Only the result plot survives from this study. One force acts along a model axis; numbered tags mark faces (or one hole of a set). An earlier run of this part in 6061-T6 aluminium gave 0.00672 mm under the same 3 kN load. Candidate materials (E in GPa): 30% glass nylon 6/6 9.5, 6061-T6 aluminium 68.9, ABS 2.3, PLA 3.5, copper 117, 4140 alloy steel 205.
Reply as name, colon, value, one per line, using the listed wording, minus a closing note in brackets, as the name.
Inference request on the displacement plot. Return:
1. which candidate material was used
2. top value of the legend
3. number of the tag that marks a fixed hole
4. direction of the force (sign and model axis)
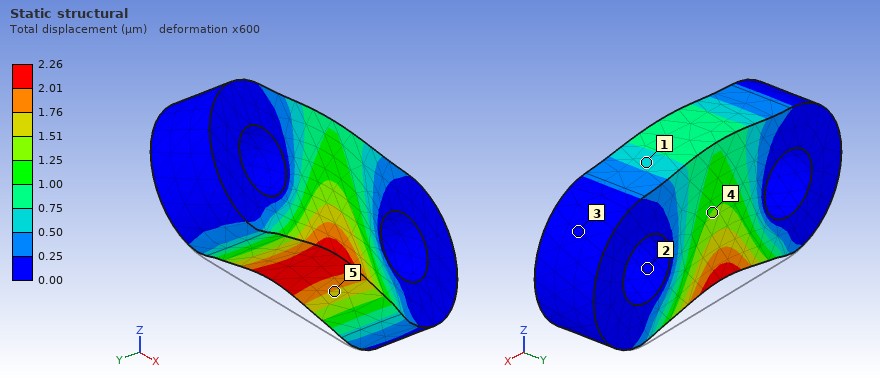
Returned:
which candidate material was used: 4140 alloy steel
top value of the legend: 2.26 µm
number of the tag that marks a fixed hole: 2
direction of the force: +Z
